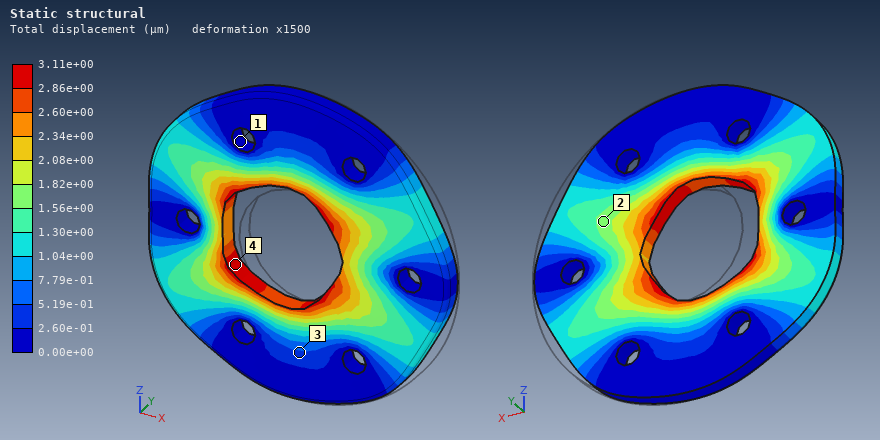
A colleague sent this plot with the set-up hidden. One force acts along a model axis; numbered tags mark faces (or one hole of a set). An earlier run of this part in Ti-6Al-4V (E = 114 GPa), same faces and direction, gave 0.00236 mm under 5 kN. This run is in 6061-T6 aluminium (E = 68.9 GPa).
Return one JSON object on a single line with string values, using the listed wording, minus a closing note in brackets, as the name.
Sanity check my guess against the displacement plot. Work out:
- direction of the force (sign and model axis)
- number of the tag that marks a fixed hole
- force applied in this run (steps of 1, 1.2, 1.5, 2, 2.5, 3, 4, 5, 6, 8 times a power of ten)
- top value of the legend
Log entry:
{"direction of the force": "-X", "number of the tag that marks a fixed hole": "1", "force applied in this run": "4 kN", "top value of the legend": "3.11e+00 µm"}
